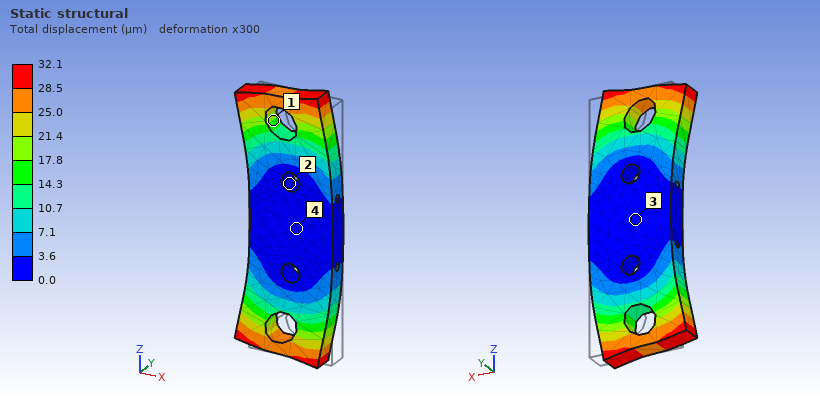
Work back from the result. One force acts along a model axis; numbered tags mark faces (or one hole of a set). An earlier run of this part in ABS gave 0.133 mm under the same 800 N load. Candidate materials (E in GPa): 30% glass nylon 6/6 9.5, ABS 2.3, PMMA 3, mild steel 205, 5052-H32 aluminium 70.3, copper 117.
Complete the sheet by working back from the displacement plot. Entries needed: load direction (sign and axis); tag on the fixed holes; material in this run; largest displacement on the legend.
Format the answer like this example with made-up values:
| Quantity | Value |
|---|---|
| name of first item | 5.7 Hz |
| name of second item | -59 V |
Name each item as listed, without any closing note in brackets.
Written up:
| Quantity | Value |
|---|---|
| load direction | -X |
| tag on the fixed holes | 2 |
| material in this run | 30% glass nylon 6/6 |
| largest displacement on the legend | 32.1 µm |
